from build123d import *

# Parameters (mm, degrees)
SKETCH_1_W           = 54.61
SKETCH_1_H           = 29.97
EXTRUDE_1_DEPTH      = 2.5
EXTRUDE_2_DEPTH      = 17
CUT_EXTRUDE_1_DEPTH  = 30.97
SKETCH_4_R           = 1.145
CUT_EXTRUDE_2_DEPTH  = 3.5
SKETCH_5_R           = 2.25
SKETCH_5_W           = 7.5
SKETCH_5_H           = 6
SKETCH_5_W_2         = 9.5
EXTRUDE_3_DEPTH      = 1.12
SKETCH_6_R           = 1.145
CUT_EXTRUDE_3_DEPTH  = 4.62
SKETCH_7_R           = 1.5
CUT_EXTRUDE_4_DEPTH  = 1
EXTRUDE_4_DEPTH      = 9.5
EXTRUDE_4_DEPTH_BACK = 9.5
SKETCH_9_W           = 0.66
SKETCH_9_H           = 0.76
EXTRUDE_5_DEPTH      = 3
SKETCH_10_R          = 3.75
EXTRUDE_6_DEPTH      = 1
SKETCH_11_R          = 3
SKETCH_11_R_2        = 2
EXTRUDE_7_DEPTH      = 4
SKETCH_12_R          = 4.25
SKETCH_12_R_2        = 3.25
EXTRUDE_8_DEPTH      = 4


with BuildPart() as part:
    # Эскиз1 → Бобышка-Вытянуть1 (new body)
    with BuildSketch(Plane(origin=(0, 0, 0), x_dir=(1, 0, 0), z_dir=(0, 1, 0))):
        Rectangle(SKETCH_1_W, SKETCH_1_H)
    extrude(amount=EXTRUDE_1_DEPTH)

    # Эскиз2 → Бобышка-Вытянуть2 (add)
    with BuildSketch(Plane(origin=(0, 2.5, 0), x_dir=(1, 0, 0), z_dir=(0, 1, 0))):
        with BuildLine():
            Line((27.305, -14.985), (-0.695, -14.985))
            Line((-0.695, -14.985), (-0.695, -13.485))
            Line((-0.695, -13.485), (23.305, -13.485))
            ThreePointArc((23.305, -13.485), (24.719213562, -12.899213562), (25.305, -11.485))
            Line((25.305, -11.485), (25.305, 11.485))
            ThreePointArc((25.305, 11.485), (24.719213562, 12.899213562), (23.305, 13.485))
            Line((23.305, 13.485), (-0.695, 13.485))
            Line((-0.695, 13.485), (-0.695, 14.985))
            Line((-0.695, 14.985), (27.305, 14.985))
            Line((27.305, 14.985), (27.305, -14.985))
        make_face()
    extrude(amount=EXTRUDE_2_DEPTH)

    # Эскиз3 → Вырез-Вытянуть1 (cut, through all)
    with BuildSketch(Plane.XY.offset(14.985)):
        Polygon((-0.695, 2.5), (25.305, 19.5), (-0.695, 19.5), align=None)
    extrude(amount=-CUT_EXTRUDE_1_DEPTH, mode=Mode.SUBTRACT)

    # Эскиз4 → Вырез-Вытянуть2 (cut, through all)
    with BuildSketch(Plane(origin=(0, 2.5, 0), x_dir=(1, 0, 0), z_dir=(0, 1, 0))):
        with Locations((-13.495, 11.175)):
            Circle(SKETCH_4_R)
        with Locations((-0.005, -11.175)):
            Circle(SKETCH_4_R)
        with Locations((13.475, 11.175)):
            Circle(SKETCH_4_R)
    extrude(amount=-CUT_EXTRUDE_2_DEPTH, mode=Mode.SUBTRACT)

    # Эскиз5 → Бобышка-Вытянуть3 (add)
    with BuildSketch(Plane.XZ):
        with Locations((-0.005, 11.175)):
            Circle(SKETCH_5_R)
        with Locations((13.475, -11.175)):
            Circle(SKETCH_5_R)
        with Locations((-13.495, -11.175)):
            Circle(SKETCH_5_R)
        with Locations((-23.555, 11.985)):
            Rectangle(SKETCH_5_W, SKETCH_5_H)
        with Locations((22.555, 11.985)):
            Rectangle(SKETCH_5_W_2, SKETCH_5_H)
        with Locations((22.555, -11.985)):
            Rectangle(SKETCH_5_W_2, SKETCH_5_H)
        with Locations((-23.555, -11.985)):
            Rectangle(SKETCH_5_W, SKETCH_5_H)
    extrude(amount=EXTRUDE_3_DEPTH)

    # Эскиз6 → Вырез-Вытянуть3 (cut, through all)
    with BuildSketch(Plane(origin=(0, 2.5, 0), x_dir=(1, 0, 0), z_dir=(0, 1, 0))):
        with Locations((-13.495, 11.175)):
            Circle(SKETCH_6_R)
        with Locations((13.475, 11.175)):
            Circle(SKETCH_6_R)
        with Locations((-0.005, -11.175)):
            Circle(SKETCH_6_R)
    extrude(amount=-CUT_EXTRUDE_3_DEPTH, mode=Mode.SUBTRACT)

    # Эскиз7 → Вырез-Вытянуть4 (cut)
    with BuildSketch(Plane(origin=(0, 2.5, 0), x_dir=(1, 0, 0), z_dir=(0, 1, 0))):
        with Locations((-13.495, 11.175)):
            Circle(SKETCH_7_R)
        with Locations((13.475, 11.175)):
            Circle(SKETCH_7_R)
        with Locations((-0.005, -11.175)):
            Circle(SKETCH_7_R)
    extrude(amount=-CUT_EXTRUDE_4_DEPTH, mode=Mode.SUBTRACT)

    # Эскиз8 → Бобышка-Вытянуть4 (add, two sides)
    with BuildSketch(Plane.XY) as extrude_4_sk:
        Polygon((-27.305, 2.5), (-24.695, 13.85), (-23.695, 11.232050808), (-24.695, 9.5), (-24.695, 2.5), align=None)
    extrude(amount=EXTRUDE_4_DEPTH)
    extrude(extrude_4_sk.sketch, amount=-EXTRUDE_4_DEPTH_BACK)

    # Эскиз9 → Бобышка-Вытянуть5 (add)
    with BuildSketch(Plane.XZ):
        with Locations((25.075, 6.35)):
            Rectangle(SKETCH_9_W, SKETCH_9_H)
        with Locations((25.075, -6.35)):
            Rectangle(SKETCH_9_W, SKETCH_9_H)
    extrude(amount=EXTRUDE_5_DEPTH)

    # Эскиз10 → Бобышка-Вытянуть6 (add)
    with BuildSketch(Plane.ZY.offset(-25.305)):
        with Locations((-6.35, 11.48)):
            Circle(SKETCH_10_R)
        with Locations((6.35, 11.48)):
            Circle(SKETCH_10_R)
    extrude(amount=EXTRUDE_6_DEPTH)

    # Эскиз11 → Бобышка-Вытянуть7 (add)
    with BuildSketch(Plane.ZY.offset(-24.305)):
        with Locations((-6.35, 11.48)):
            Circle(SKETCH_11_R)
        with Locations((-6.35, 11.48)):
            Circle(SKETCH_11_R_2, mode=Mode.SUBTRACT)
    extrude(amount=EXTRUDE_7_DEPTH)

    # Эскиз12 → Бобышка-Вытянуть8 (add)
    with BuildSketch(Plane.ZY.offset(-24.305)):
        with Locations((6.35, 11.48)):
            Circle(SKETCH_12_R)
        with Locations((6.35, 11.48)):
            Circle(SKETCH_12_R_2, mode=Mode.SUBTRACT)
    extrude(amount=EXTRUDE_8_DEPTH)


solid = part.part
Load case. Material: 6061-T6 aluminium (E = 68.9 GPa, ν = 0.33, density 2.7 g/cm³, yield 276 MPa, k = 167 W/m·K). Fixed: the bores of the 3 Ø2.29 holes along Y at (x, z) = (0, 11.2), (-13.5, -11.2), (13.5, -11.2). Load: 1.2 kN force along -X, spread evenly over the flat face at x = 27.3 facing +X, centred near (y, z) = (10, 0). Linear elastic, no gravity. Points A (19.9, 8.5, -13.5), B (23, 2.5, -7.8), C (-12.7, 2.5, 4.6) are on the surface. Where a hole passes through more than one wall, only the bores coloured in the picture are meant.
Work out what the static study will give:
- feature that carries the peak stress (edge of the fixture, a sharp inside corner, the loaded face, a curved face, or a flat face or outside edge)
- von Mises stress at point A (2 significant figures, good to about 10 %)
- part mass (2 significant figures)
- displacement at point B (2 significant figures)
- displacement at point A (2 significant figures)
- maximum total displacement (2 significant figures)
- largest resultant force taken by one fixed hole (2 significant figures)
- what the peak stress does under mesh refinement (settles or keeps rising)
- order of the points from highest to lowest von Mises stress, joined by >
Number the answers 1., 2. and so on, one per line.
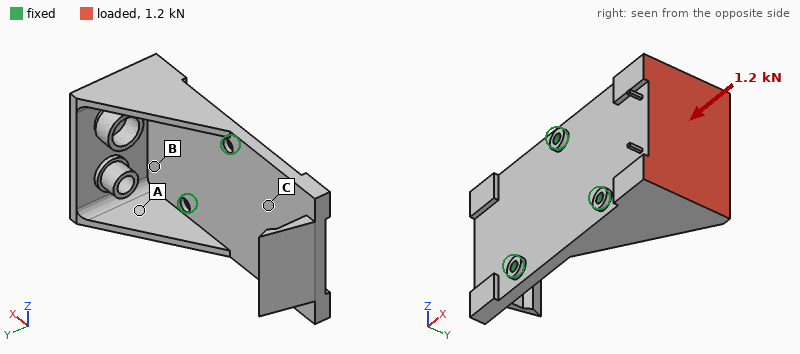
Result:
1. edge of the fixture
2. 70 MPa
3. 18 g
4. 0.095 mm
5. 0.095 mm
6. 0.41 mm
7. 580 N
8. keeps rising
9. A > B > C
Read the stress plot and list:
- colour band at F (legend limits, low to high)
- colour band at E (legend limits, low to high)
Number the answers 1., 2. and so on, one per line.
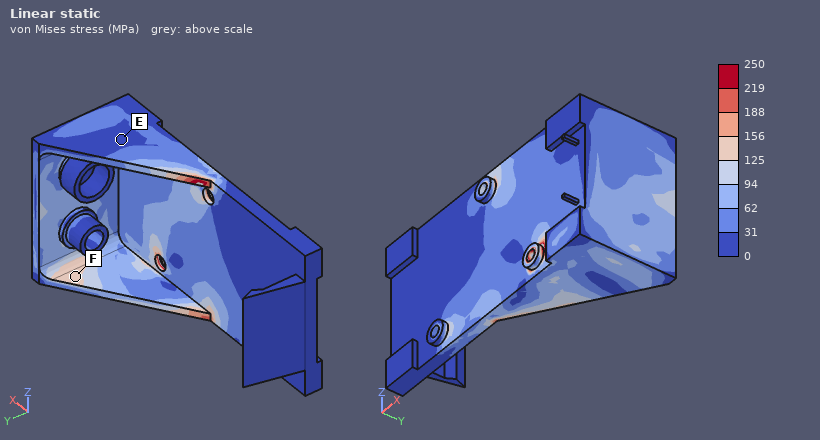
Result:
1. 125 to 156 MPa
2. 0 to 31 MPa
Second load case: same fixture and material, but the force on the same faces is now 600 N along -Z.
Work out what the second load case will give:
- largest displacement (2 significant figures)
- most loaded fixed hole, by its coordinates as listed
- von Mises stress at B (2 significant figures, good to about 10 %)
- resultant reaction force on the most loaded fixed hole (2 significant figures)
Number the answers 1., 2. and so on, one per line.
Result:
1. 0.29 mm
2. (13.5, -11.2)
3. 62 MPa
4. 610 N
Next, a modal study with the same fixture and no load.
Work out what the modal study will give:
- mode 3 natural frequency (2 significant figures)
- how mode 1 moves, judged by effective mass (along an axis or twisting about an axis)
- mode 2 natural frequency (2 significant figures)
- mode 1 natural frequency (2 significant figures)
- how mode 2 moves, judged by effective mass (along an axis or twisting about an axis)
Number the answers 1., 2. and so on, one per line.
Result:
1. 5900 Hz
2. along Y
3. 3400 Hz
4. 2500 Hz
5. along Y
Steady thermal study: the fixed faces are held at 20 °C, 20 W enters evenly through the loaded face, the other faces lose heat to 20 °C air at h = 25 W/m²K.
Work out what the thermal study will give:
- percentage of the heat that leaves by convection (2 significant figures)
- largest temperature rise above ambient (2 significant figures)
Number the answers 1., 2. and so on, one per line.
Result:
1. 8.1 %
2. 31 K
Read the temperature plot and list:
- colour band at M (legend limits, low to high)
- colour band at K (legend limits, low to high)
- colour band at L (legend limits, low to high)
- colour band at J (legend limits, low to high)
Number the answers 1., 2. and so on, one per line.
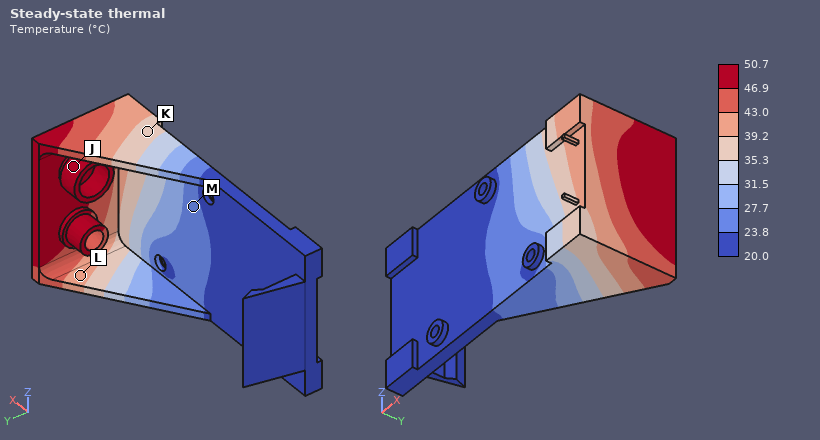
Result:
1. 23.8 to 27.7 °C
2. 35.3 to 39.2 °C
3. 39.2 to 43.0 °C
4. 46.9 to 50.7 °C
